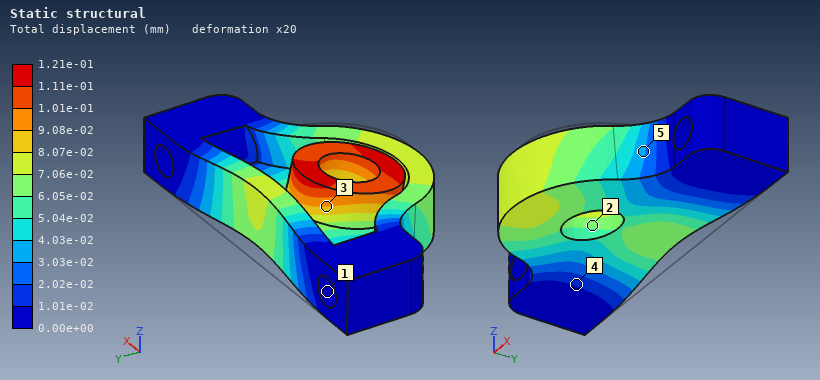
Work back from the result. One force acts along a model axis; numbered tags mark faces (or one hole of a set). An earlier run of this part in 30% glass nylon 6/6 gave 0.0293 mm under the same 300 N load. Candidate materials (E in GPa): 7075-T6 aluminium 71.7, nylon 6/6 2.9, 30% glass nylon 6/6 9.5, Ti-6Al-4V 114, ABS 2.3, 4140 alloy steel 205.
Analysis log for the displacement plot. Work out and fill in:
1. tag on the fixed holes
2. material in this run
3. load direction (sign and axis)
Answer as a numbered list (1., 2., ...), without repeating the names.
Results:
1. 1
2. ABS
3. -Y
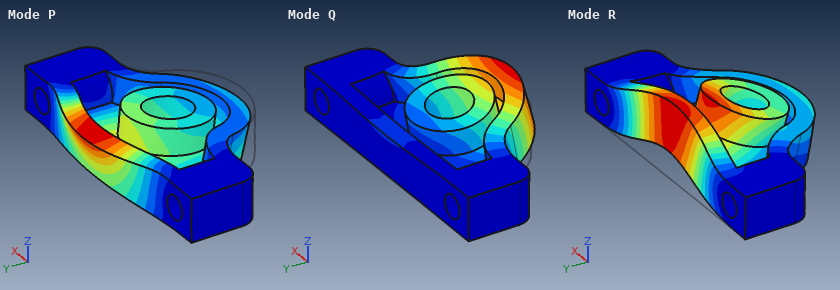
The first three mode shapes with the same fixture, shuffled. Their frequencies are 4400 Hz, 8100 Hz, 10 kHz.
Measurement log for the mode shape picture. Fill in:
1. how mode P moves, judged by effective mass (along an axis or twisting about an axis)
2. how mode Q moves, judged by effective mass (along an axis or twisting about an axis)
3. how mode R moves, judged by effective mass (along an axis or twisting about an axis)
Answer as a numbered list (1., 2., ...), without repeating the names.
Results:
1. along Y
2. along Z
3. along Z
